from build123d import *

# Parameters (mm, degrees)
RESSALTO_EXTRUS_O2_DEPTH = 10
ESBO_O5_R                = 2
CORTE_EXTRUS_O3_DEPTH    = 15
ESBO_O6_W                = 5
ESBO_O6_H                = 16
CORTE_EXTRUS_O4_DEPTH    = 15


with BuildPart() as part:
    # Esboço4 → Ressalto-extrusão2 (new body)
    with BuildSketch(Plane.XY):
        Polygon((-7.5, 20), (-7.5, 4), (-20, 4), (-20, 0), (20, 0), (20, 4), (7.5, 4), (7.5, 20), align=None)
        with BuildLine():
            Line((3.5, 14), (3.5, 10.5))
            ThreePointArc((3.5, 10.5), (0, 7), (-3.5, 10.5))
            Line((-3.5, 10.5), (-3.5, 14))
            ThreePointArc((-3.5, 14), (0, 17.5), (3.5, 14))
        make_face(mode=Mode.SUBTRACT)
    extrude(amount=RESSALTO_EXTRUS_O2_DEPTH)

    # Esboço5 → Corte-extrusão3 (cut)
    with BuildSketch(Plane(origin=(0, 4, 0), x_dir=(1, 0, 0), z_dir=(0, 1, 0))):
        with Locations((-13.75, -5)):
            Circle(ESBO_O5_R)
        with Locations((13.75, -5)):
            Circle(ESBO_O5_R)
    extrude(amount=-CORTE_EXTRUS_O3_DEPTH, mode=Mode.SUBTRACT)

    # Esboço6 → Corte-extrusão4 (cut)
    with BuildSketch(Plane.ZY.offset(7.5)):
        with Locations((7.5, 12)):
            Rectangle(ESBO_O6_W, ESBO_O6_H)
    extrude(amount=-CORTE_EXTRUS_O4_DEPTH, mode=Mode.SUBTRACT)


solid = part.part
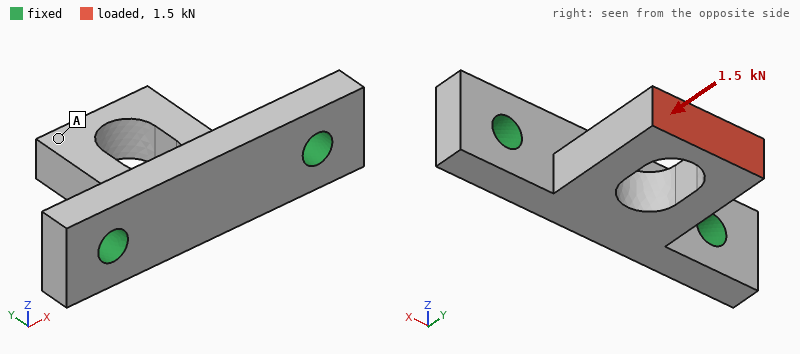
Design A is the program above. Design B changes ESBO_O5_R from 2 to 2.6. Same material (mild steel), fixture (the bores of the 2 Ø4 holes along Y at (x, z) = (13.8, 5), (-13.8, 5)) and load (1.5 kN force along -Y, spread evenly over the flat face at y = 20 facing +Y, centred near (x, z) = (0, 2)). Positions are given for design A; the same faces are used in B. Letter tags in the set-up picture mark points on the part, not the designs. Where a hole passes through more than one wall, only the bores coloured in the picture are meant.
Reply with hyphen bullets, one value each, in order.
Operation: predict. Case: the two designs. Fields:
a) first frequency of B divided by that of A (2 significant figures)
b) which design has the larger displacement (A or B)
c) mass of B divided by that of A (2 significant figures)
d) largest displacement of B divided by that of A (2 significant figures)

- 1.0
- A
- 0.97
- 0.86
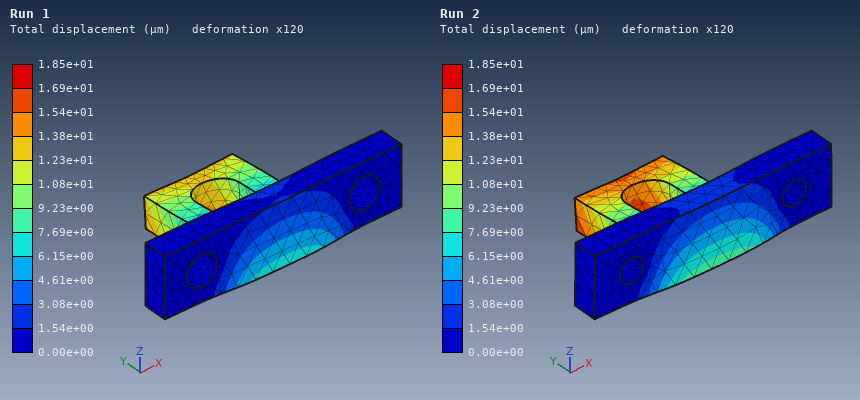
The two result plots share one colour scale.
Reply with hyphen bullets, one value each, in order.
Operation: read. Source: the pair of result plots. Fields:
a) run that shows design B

- Run 1
